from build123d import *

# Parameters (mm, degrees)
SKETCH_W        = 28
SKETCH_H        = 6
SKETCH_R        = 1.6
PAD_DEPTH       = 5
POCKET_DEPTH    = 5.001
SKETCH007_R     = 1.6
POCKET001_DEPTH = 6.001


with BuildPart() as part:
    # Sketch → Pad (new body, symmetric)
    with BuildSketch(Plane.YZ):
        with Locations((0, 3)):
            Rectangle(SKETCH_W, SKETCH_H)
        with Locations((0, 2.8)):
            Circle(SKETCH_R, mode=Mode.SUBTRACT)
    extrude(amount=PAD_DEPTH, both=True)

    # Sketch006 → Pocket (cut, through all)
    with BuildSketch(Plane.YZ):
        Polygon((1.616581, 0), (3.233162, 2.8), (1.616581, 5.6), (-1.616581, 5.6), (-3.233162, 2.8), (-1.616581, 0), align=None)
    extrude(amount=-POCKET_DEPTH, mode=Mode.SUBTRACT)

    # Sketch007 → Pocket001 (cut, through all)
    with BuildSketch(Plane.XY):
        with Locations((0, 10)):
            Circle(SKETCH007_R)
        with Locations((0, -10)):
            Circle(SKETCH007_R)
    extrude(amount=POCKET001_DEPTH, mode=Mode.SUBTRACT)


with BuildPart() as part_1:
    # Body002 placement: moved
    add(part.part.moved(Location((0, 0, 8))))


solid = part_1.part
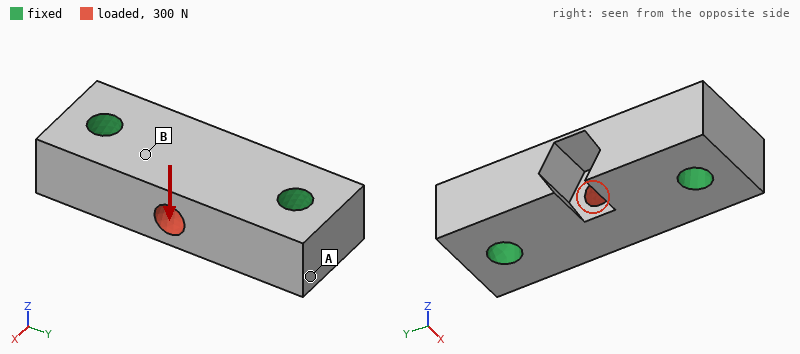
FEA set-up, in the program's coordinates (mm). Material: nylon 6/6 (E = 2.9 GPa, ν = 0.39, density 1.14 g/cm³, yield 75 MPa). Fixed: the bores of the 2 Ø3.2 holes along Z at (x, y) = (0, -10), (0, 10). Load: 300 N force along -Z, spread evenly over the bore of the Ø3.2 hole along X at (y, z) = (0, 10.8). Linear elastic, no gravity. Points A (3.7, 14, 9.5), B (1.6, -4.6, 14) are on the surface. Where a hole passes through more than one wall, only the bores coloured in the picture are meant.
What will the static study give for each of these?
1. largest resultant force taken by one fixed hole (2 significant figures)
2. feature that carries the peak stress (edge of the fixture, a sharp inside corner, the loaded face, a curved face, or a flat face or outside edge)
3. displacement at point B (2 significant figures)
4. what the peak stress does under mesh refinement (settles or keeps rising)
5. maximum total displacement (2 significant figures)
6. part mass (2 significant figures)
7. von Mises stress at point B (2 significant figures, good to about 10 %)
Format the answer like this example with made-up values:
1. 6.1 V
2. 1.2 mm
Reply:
1. 150 N
2. edge of the fixture
3. 38 µm
4. keeps rising
5. 90 µm
6. 1.6 g
7. 5.7 MPa
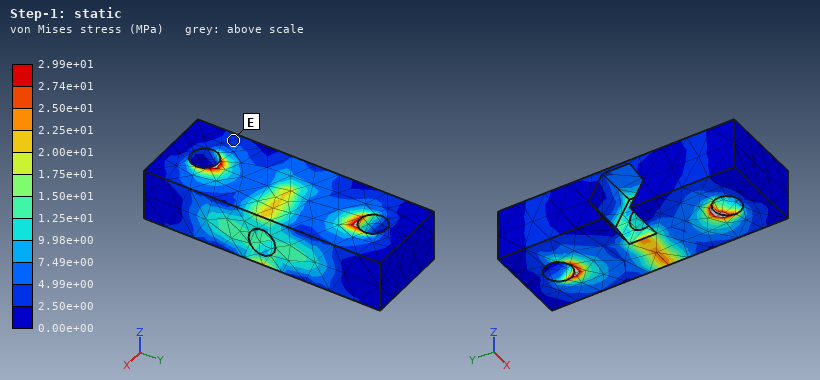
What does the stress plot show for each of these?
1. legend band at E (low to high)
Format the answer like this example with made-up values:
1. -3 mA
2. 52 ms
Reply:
1. 2.50e+00 to 4.99e+00 MPa
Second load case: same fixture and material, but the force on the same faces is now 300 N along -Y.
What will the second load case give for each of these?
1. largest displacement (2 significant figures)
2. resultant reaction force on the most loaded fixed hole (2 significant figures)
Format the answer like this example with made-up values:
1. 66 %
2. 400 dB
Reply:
1. 17 µm
2. 150 N
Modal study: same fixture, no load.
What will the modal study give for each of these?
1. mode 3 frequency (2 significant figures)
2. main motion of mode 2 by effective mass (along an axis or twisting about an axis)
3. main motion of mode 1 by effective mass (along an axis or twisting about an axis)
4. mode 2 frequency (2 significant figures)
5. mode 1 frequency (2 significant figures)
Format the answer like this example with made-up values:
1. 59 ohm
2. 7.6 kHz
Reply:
1. 24 kHz
2. along Z
3. along X
4. 19 kHz
5. 18 kHz
